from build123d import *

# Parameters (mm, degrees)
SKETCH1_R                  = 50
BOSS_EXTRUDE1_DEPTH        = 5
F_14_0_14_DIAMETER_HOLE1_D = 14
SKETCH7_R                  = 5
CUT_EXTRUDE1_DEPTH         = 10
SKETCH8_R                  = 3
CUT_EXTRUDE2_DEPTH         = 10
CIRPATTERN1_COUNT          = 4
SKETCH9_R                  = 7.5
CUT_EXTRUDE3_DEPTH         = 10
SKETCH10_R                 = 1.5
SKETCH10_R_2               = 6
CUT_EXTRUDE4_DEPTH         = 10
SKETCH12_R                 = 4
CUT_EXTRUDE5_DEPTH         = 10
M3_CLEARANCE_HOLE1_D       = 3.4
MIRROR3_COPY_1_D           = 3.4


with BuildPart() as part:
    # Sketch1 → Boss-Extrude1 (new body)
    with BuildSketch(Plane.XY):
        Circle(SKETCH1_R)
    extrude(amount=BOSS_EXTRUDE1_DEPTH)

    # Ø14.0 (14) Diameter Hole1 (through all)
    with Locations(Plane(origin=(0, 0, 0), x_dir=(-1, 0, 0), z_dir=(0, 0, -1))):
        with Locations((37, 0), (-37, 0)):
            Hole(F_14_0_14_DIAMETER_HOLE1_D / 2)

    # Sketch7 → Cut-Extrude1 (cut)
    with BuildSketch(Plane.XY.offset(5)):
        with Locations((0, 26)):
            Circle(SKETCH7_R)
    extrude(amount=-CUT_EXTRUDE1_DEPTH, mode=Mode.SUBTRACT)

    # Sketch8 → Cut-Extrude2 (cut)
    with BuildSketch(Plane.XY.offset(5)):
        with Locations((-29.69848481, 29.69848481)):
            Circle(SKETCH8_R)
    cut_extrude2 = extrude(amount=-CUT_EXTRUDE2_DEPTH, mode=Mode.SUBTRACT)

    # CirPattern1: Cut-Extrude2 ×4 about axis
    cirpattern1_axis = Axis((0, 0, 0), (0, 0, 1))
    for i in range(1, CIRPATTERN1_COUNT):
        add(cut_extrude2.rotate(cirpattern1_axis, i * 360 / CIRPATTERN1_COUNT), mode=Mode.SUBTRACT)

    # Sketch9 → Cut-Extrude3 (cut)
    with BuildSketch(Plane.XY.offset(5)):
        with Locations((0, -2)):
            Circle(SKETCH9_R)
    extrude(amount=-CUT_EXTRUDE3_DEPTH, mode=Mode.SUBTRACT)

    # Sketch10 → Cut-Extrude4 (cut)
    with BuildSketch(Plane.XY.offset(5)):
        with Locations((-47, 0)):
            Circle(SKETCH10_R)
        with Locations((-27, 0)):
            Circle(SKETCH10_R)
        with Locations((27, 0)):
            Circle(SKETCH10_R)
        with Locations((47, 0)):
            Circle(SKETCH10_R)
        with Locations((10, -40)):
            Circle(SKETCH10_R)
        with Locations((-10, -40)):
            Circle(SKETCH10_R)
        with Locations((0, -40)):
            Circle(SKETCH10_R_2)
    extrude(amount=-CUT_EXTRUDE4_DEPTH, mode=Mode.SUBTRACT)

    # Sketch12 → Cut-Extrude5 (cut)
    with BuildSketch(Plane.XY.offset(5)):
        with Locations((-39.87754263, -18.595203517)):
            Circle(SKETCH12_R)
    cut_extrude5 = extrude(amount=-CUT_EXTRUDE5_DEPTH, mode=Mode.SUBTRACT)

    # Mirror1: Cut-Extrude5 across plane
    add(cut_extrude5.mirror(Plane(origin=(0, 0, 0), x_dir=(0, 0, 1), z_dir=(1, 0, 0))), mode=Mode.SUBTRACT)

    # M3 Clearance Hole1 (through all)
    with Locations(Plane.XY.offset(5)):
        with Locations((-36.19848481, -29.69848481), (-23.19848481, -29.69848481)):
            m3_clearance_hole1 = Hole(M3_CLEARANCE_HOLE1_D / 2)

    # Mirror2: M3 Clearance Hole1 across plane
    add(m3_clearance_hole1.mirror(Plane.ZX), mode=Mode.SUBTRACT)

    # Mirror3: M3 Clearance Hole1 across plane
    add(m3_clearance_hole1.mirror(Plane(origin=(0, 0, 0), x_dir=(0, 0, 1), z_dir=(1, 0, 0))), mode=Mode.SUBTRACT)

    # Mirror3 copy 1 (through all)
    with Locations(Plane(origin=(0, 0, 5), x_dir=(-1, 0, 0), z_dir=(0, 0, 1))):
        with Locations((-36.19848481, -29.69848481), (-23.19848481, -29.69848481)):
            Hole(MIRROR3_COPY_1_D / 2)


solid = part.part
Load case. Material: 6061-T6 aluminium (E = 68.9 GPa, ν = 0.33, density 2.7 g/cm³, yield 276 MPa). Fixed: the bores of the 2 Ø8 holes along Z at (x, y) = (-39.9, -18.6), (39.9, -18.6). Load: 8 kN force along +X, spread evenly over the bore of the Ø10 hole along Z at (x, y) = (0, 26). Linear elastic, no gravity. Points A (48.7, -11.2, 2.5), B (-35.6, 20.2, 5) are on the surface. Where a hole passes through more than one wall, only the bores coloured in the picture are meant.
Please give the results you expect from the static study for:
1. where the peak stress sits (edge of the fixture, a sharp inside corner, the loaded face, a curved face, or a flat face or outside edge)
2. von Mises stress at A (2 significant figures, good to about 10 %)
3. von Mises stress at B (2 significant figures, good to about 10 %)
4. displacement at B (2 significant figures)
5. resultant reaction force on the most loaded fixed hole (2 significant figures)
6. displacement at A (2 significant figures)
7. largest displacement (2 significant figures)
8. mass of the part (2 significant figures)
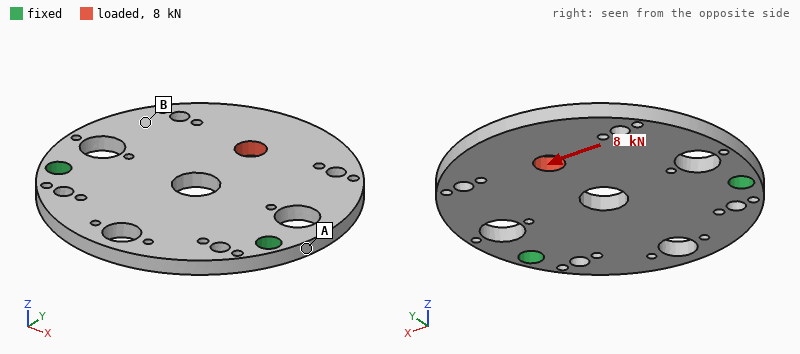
a curved face
67 MPa
19 MPa
60 µm
5.9 kN
16 µm
83 µm
92 g
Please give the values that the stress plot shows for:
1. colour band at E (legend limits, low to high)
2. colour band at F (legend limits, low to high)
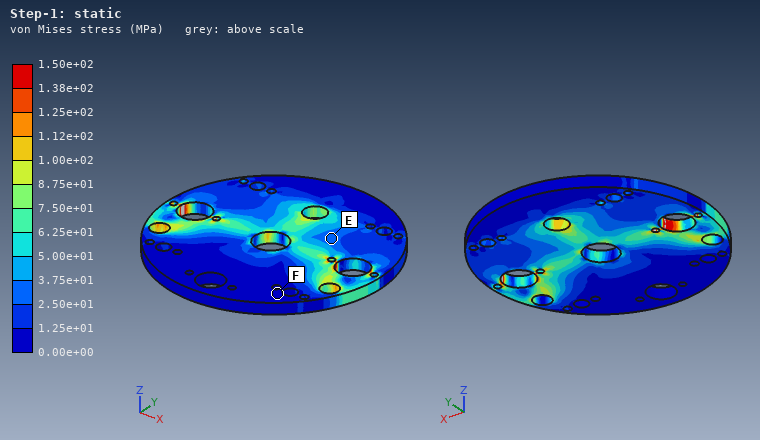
2.50e+01 to 3.75e+01 MPa
0.00e+00 to 1.25e+01 MPa
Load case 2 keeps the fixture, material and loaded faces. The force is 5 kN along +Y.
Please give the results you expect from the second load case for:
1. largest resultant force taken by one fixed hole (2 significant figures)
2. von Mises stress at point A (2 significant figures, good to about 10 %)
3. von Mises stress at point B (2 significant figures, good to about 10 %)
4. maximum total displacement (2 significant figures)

2.6 kN
19 MPa
6.0 MPa
28 µm
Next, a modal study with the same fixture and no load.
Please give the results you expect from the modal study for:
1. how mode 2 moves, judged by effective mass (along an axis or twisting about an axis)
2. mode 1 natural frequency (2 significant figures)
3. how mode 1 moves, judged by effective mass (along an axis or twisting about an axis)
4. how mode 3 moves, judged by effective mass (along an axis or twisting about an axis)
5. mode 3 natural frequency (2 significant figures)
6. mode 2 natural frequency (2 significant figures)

twisting about Y
840 Hz
along Z
along Z
3000 Hz
2400 Hz
